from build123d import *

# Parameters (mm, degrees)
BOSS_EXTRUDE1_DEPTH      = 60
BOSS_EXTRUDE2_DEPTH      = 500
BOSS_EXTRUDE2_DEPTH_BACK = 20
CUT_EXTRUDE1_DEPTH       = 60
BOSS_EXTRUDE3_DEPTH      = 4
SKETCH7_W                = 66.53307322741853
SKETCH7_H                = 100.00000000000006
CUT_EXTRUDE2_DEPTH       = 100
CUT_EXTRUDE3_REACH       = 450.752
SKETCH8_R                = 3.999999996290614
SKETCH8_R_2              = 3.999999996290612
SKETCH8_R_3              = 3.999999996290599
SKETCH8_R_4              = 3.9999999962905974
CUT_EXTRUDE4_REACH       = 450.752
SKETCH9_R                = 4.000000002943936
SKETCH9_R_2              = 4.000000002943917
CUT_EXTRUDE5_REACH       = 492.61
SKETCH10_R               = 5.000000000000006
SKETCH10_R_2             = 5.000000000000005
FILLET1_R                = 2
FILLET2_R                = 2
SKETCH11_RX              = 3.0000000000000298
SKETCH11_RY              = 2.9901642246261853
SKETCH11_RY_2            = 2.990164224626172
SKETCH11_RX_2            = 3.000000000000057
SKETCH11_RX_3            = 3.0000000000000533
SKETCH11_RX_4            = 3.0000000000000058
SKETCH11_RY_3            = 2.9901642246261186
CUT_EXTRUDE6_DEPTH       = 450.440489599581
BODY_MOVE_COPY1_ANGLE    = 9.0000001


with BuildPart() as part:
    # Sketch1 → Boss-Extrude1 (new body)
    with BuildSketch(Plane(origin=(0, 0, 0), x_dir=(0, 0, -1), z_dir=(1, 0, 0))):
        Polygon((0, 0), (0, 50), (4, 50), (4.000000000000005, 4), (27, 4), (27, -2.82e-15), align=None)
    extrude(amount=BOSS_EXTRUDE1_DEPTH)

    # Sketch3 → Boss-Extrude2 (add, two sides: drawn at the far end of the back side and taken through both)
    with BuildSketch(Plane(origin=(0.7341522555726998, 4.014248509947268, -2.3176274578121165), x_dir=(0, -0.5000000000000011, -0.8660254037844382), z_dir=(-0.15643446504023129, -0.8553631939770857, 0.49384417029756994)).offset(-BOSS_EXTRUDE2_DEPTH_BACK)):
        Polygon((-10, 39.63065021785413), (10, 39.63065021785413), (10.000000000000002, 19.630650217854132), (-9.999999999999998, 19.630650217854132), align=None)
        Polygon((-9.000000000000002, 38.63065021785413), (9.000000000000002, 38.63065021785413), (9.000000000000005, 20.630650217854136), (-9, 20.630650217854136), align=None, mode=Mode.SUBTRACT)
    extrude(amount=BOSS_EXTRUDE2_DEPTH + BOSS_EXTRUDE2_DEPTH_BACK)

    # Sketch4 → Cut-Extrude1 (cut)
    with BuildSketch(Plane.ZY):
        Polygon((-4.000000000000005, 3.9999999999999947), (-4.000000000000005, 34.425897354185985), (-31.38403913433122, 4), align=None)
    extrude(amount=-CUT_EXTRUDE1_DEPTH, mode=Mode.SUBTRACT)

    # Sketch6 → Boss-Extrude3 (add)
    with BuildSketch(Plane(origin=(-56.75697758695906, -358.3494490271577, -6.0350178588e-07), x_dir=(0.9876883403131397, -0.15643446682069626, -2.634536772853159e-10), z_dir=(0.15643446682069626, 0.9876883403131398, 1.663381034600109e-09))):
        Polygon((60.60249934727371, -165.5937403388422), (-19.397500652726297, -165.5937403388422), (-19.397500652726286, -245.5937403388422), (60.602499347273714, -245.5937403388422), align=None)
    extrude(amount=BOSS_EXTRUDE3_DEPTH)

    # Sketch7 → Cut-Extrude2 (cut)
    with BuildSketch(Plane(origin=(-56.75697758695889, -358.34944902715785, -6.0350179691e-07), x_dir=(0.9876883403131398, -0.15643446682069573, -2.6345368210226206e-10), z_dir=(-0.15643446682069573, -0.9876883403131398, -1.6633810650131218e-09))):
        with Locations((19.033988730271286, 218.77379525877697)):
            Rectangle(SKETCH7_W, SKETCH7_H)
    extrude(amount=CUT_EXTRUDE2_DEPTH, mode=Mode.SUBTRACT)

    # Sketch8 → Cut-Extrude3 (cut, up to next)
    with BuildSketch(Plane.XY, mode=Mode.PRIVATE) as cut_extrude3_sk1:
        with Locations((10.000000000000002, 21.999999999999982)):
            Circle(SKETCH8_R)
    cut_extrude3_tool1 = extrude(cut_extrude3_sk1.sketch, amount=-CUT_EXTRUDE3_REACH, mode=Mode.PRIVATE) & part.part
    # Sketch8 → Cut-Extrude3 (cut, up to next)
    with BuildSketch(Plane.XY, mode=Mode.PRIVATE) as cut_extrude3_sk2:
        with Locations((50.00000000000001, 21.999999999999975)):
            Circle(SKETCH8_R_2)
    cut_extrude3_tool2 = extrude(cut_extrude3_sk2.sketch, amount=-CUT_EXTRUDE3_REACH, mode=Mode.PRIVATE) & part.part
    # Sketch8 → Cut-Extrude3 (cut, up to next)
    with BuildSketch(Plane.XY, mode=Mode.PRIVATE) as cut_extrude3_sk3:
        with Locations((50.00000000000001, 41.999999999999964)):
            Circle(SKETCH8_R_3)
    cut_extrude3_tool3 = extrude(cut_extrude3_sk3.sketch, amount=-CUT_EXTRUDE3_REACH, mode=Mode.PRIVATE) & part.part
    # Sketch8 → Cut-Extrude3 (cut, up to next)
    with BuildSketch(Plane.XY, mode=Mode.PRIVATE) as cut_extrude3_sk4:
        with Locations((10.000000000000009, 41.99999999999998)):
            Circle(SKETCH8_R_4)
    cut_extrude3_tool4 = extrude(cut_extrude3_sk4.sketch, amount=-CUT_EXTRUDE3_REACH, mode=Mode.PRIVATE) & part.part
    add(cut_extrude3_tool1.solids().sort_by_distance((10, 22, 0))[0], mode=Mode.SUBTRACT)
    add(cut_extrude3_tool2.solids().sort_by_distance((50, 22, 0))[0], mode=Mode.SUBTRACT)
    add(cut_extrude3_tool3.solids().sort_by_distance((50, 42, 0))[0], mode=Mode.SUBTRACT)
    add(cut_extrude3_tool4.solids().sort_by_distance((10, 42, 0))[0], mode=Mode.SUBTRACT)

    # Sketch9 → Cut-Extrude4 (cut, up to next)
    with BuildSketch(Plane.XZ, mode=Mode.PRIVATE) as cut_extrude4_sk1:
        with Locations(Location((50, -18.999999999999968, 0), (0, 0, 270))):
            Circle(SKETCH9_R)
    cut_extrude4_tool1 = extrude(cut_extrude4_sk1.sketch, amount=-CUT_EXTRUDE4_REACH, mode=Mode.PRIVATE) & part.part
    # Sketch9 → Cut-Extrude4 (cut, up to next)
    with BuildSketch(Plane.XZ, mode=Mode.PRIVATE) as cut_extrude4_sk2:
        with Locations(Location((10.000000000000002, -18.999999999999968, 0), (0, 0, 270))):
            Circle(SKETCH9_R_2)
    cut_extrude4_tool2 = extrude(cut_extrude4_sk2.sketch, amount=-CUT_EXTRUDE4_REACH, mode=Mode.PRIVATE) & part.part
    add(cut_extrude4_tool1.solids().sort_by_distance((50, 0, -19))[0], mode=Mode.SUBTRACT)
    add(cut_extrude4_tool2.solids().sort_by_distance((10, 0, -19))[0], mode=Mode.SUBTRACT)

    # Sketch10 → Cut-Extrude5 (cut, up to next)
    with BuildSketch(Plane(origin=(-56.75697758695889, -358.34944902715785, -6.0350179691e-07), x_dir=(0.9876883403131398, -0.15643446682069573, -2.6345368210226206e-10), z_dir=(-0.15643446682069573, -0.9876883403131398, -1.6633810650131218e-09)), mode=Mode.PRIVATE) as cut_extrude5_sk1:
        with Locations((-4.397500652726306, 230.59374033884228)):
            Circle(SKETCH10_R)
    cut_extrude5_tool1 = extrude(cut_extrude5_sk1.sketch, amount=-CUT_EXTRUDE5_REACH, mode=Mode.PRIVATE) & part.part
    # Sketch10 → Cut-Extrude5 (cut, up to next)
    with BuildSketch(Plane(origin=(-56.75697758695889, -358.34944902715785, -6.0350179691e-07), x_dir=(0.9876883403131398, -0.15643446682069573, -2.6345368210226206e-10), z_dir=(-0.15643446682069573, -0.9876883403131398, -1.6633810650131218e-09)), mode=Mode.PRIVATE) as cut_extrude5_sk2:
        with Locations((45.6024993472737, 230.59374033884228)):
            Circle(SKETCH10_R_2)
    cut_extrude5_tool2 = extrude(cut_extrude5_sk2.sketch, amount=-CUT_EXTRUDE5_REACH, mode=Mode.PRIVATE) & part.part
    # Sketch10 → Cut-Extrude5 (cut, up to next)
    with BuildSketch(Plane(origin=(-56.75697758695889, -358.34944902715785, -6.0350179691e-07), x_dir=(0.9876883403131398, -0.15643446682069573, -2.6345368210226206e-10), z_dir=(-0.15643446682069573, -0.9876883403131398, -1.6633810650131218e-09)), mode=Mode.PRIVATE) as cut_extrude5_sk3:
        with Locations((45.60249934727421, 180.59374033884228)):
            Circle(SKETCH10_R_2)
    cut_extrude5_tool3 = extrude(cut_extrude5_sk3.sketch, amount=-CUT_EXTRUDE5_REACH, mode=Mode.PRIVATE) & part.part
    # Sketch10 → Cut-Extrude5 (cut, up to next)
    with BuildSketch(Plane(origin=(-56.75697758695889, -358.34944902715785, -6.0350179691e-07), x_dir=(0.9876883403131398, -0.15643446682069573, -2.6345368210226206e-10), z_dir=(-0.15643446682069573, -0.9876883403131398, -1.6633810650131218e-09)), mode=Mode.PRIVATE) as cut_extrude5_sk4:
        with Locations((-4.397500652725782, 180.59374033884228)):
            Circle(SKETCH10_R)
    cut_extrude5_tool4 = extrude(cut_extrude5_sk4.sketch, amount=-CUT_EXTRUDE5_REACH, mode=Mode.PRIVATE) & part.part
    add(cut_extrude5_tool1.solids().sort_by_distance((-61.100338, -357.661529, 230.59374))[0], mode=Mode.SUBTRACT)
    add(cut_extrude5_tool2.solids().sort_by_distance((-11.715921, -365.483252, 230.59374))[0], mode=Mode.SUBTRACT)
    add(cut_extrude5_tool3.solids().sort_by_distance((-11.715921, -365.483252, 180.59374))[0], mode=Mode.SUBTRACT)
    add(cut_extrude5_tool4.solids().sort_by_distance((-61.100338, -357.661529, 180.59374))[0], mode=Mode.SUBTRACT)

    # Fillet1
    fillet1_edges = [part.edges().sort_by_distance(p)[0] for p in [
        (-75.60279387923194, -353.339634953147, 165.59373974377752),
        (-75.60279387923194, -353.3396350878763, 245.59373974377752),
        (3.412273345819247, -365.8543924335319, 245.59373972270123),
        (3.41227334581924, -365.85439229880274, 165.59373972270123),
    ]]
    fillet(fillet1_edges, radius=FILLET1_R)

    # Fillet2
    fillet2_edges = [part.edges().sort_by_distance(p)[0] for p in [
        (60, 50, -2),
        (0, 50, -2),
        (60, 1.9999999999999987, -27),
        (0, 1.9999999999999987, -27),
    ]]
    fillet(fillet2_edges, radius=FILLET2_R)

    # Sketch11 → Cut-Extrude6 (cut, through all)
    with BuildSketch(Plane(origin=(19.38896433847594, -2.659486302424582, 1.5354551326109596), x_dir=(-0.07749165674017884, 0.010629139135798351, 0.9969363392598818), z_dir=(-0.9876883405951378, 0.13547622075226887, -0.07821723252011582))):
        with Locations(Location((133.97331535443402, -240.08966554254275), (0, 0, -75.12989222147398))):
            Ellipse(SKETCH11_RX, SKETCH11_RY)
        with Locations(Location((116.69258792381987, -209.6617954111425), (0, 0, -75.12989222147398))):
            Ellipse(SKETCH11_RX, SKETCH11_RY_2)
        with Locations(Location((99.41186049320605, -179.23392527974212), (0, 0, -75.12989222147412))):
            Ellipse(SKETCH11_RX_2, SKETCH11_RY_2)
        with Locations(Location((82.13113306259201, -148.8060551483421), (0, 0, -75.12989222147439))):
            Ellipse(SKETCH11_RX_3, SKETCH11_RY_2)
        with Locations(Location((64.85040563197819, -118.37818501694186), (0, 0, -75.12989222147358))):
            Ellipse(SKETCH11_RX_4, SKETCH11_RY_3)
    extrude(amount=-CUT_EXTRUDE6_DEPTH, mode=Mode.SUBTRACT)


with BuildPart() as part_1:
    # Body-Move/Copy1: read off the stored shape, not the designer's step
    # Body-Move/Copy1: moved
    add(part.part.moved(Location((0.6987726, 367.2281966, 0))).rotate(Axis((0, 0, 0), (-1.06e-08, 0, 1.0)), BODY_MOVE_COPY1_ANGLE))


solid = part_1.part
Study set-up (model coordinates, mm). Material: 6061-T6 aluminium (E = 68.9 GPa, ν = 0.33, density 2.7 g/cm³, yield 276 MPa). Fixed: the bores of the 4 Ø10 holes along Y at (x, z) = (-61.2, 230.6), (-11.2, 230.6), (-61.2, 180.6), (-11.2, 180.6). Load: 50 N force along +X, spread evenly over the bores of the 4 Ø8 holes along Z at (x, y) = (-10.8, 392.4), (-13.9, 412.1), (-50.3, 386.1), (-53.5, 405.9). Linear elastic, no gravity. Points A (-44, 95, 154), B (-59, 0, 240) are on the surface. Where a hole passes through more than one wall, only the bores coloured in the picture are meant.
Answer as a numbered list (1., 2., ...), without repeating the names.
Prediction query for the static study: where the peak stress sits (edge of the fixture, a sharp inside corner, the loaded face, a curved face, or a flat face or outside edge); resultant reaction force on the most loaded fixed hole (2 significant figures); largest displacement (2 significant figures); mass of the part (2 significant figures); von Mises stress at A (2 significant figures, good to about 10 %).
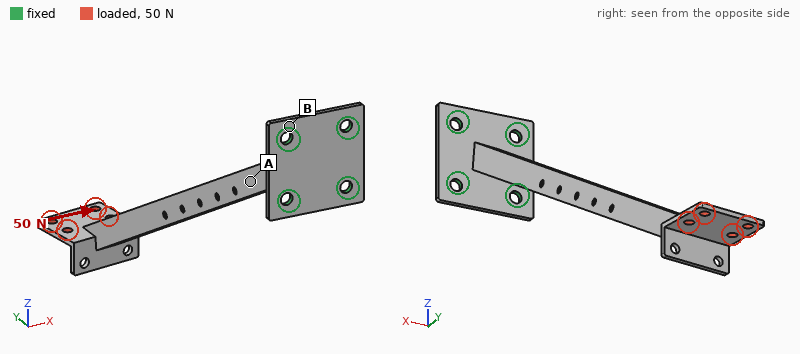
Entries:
1. a curved face
2. 300 N
3. 6.0 mm
4. 200 g
5. 37 MPa
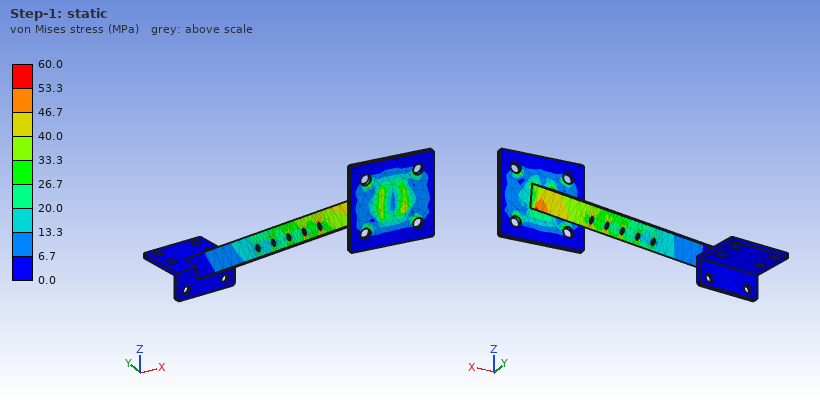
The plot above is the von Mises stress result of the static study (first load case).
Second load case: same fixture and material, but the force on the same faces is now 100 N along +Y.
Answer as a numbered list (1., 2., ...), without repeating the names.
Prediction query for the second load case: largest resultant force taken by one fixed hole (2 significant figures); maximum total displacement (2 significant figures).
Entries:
1. 310 N
2. 5.3 mm
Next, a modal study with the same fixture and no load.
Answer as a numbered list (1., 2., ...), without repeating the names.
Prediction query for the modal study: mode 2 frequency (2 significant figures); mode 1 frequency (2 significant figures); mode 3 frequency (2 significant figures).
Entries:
1. 62 Hz
2. 62 Hz
3. 490 Hz
